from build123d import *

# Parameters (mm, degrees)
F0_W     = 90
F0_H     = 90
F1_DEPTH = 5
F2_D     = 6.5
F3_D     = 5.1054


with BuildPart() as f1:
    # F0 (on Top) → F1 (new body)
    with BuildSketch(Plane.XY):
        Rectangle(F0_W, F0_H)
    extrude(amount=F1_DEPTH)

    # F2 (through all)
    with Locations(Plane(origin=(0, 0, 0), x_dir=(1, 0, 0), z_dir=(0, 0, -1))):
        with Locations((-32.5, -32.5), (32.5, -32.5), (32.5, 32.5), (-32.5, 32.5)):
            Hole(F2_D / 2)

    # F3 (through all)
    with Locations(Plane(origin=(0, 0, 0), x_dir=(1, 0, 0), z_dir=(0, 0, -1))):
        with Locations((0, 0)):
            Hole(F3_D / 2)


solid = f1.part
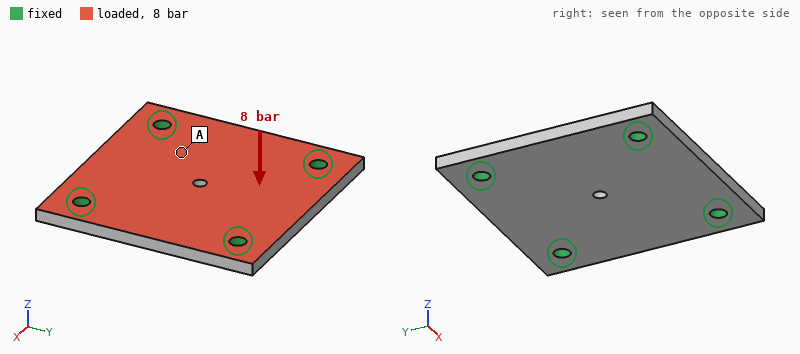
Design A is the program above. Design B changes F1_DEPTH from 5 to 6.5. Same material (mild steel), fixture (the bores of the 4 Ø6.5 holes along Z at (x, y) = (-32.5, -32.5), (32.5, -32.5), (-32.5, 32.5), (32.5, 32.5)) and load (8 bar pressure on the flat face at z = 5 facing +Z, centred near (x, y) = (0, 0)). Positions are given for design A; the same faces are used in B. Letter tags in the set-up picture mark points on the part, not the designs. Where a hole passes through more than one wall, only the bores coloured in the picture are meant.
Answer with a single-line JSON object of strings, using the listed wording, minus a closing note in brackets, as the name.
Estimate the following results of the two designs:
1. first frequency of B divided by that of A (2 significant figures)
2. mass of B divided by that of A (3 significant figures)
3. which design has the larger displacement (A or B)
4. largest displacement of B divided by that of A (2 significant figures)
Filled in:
{"first frequency of B divided by that of A": "1.2", "mass of B divided by that of A": "1.30", "which design has the larger displacement": "A", "largest displacement of B divided by that of A": "0.49"}
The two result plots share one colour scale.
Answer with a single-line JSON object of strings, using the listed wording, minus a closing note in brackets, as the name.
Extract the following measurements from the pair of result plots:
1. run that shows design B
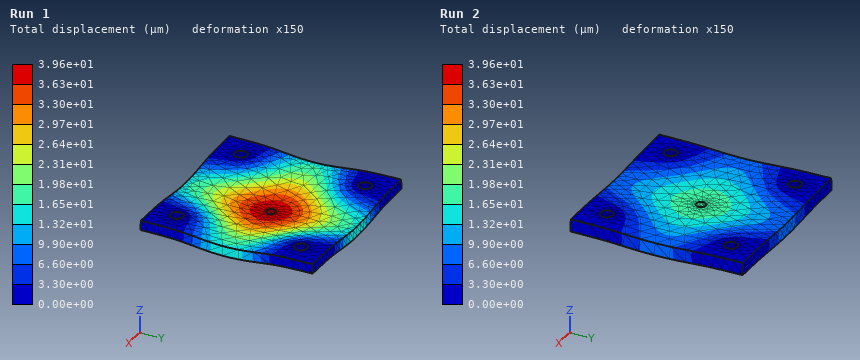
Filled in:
{"run that shows design B": "Run 2"}
